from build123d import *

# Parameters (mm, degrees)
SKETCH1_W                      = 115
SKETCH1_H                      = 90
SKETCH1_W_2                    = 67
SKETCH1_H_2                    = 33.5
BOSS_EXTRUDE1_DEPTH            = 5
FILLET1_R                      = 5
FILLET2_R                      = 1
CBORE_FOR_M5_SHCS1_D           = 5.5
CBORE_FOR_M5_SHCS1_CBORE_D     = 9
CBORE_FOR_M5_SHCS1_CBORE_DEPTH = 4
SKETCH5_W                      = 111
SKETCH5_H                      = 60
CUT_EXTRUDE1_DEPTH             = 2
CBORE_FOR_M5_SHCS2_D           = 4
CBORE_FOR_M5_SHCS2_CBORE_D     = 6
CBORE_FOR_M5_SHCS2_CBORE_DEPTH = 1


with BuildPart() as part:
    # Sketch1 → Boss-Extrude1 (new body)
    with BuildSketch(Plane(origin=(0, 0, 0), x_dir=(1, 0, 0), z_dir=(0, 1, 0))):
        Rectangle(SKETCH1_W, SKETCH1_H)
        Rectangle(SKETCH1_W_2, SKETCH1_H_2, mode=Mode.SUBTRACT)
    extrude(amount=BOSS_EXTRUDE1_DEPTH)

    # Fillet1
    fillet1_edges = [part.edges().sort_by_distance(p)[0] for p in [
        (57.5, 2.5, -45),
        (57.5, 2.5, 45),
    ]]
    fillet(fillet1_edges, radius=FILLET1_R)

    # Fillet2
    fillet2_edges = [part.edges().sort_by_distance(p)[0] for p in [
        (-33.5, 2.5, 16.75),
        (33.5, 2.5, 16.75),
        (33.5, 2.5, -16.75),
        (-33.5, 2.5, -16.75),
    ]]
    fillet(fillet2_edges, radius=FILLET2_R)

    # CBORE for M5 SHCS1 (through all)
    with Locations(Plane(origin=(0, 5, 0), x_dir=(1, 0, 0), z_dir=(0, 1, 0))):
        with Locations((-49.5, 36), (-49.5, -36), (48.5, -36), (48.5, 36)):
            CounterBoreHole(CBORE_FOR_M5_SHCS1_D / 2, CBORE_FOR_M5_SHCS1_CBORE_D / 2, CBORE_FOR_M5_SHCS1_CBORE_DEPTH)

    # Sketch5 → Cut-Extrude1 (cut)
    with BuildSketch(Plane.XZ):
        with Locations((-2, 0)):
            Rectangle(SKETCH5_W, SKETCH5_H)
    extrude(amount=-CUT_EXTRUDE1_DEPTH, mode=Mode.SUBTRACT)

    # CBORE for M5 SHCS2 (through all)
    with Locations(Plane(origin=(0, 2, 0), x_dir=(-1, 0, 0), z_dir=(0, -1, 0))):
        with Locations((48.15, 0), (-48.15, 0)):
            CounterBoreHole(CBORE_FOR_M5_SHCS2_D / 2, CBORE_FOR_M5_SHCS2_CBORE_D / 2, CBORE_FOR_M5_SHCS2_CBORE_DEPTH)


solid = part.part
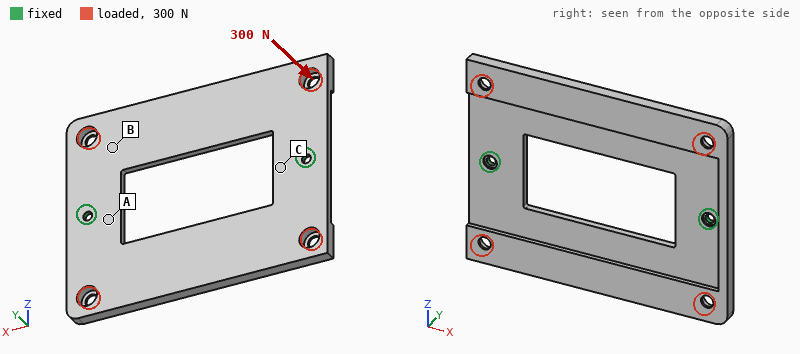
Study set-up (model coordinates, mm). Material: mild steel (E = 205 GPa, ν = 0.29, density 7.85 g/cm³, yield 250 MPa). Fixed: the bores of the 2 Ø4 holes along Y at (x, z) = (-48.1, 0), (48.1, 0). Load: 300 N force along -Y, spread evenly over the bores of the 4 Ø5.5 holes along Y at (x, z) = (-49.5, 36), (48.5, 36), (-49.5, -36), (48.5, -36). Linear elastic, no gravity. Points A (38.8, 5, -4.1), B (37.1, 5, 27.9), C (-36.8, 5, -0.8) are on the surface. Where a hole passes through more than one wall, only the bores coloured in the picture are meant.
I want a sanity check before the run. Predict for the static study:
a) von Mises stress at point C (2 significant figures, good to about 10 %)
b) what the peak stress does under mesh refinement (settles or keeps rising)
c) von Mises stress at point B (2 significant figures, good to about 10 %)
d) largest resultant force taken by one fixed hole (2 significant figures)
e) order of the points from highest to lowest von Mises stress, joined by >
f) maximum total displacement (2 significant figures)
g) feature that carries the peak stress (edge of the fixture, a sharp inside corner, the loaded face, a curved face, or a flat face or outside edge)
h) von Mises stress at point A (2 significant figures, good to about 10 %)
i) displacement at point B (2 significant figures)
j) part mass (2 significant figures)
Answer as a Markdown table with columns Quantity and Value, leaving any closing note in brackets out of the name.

| Quantity | Value |
|---|---|
| von Mises stress at point C | 59 MPa |
| what the peak stress does under mesh refinement | keeps rising |
| von Mises stress at point B | 10 MPa |
| largest resultant force taken by one fixed hole | 170 N |
| order of the points from highest to lowest von Mises stress, joined by > | C > A > B |
| maximum total displacement | 0.12 mm |
| feature that carries the peak stress | edge of the fixture |
| von Mises stress at point A | 44 MPa |
| displacement at point B | 0.046 mm |
| part mass | 240 g |
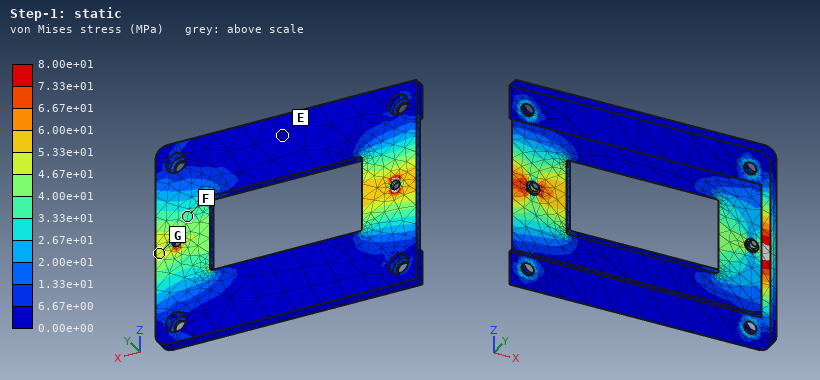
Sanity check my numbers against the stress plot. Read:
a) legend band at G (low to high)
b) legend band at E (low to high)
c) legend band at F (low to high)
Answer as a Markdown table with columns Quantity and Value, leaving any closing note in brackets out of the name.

| Quantity | Value |
|---|---|
| legend band at G | 4.67e+01 to 5.33e+01 MPa |
| legend band at E | 0.00e+00 to 6.67e+00 MPa |
| legend band at F | 3.33e+01 to 4.00e+01 MPa |
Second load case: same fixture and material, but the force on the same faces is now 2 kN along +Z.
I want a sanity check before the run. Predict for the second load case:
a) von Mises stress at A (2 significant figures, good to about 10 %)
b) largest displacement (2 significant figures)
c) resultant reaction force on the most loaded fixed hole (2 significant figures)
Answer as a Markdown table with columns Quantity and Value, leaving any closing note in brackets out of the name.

| Quantity | Value |
|---|---|
| von Mises stress at A | 23 MPa |
| largest displacement | 0.14 mm |
| resultant reaction force on the most loaded fixed hole | 1.0 kN |
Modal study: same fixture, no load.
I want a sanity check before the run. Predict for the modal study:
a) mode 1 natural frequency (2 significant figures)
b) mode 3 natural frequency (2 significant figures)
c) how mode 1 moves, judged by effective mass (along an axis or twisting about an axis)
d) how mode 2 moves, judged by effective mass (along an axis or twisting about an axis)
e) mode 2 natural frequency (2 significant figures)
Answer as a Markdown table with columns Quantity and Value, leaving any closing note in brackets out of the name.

| Quantity | Value |
|---|---|
| mode 1 natural frequency | 550 Hz |
| mode 3 natural frequency | 1400 Hz |
| how mode 1 moves, judged by effective mass | twisting about X |
| how mode 2 moves, judged by effective mass | along Y |
| mode 2 natural frequency | 700 Hz |
